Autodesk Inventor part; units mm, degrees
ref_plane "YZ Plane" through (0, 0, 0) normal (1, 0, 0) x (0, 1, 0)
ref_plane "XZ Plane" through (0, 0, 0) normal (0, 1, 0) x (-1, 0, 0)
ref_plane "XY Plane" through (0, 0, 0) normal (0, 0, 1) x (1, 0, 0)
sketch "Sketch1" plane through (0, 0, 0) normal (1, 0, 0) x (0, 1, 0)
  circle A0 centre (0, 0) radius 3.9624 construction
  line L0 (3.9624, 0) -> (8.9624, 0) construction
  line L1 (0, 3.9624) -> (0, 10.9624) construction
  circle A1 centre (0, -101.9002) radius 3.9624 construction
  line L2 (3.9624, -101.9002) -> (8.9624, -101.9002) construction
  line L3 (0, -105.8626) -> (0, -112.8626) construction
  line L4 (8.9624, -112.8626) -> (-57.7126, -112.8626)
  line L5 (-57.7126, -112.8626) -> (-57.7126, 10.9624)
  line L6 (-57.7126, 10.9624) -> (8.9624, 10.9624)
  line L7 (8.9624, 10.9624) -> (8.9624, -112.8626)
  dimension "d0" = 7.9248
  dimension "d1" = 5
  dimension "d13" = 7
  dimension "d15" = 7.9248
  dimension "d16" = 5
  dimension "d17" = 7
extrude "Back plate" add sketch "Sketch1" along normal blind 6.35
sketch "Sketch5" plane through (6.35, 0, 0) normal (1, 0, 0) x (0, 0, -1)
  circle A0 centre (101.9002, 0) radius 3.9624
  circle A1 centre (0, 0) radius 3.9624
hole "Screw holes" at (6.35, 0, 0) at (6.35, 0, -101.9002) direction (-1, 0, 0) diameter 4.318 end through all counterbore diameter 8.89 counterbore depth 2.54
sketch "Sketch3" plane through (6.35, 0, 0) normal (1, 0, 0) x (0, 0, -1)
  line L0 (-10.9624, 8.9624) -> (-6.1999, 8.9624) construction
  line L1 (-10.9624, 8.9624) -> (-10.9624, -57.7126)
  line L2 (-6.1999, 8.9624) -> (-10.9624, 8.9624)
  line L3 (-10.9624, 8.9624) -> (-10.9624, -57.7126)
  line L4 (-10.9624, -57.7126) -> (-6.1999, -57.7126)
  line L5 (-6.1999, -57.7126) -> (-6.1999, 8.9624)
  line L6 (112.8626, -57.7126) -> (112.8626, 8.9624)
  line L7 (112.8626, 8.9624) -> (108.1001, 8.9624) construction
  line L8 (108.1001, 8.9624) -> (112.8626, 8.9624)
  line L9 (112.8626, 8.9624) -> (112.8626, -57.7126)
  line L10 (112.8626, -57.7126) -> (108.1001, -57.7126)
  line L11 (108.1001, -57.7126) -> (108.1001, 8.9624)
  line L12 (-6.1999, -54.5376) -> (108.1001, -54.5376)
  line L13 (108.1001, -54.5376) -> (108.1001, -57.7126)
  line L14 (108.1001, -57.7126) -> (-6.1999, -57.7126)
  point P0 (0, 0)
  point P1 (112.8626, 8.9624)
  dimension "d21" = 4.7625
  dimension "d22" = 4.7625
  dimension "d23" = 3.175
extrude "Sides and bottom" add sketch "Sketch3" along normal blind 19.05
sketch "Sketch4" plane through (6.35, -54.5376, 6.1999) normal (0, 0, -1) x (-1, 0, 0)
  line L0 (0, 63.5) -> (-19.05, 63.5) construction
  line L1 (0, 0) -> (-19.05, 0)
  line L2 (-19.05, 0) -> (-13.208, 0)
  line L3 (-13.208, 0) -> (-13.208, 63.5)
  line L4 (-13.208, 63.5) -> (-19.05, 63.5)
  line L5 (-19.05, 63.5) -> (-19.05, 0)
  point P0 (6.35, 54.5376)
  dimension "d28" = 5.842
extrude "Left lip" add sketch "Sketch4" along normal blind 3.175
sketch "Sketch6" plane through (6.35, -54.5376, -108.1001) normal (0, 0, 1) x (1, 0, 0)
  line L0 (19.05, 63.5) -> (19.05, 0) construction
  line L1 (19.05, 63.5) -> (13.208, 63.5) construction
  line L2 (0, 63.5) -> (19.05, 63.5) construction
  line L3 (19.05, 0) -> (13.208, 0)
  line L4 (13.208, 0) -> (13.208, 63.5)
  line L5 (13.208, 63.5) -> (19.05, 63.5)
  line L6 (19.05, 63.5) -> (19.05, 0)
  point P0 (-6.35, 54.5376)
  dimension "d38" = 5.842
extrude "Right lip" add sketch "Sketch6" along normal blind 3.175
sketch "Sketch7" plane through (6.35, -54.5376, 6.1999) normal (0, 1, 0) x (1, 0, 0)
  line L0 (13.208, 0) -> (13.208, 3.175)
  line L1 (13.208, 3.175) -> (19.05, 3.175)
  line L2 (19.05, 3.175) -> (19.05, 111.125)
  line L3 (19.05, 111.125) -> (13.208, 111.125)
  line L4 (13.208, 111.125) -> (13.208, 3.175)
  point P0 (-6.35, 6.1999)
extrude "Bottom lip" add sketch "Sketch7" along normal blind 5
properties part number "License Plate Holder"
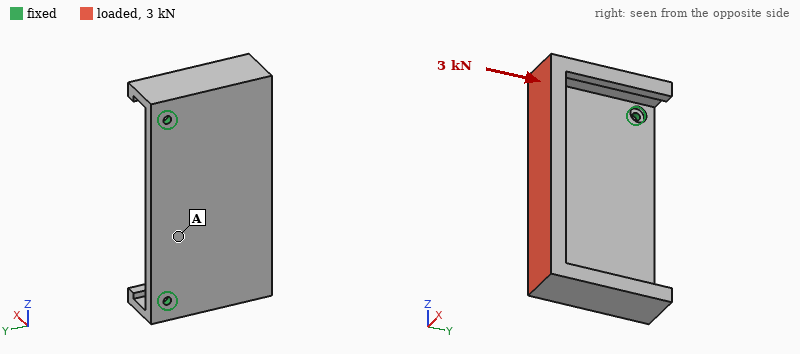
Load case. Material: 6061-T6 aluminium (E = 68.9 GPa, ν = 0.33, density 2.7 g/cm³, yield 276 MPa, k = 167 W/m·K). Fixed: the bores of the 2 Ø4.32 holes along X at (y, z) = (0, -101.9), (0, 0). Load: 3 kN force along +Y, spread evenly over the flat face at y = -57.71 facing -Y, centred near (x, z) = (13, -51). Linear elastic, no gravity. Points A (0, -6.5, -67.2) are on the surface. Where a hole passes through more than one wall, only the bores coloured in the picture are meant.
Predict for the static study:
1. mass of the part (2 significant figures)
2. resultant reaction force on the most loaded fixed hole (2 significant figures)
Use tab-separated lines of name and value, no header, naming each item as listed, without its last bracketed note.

mass of the part	210 g
resultant reaction force on the most loaded fixed hole	1.5 kN
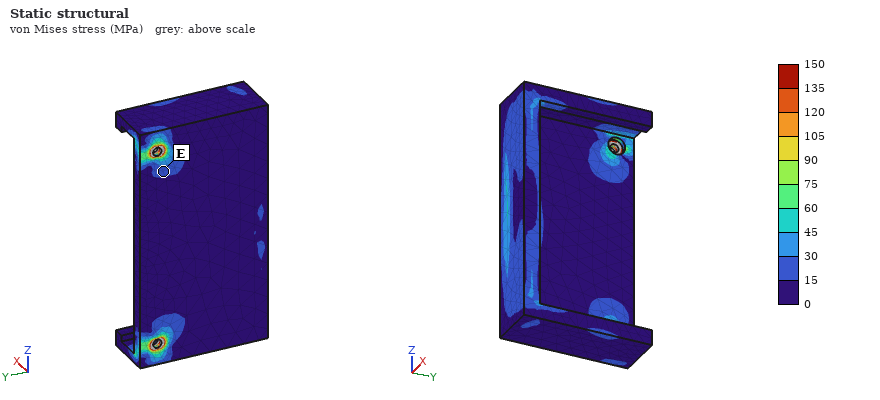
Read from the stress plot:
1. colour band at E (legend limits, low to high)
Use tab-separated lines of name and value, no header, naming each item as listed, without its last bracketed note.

colour band at E	15 to 30 MPa
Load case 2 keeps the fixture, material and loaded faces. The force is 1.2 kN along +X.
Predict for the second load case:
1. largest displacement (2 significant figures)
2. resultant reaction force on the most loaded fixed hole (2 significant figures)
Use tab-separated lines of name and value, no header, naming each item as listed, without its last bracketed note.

largest displacement	0.78 mm
resultant reaction force on the most loaded fixed hole	610 N
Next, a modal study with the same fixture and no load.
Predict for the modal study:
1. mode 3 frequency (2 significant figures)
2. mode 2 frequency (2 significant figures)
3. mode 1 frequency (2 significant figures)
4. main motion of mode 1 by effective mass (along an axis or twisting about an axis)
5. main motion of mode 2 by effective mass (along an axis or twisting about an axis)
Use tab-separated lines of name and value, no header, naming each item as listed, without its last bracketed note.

mode 3 frequency	2800 Hz
mode 2 frequency	1400 Hz
mode 1 frequency	730 Hz
main motion of mode 1 by effective mass	along X
main motion of mode 2 by effective mass	twisting about Y
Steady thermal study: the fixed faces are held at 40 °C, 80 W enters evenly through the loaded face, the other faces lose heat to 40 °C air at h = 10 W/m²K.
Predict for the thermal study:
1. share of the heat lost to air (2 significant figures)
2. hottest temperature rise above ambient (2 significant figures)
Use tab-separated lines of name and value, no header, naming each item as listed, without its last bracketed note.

share of the heat lost to air	9.8 %
hottest temperature rise above ambient	51 K
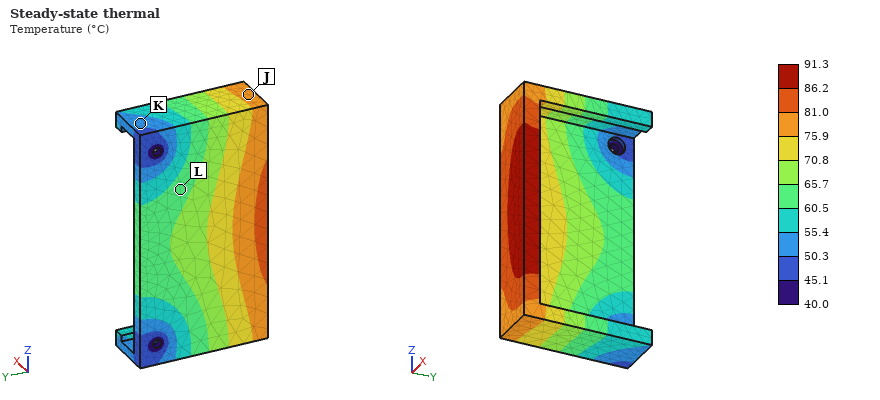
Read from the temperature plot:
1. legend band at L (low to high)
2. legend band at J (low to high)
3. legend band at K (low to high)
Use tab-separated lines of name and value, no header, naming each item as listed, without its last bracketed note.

legend band at L	60.5 to 65.7 °C
legend band at J	75.9 to 81.0 °C
legend band at K	50.3 to 55.4 °C
